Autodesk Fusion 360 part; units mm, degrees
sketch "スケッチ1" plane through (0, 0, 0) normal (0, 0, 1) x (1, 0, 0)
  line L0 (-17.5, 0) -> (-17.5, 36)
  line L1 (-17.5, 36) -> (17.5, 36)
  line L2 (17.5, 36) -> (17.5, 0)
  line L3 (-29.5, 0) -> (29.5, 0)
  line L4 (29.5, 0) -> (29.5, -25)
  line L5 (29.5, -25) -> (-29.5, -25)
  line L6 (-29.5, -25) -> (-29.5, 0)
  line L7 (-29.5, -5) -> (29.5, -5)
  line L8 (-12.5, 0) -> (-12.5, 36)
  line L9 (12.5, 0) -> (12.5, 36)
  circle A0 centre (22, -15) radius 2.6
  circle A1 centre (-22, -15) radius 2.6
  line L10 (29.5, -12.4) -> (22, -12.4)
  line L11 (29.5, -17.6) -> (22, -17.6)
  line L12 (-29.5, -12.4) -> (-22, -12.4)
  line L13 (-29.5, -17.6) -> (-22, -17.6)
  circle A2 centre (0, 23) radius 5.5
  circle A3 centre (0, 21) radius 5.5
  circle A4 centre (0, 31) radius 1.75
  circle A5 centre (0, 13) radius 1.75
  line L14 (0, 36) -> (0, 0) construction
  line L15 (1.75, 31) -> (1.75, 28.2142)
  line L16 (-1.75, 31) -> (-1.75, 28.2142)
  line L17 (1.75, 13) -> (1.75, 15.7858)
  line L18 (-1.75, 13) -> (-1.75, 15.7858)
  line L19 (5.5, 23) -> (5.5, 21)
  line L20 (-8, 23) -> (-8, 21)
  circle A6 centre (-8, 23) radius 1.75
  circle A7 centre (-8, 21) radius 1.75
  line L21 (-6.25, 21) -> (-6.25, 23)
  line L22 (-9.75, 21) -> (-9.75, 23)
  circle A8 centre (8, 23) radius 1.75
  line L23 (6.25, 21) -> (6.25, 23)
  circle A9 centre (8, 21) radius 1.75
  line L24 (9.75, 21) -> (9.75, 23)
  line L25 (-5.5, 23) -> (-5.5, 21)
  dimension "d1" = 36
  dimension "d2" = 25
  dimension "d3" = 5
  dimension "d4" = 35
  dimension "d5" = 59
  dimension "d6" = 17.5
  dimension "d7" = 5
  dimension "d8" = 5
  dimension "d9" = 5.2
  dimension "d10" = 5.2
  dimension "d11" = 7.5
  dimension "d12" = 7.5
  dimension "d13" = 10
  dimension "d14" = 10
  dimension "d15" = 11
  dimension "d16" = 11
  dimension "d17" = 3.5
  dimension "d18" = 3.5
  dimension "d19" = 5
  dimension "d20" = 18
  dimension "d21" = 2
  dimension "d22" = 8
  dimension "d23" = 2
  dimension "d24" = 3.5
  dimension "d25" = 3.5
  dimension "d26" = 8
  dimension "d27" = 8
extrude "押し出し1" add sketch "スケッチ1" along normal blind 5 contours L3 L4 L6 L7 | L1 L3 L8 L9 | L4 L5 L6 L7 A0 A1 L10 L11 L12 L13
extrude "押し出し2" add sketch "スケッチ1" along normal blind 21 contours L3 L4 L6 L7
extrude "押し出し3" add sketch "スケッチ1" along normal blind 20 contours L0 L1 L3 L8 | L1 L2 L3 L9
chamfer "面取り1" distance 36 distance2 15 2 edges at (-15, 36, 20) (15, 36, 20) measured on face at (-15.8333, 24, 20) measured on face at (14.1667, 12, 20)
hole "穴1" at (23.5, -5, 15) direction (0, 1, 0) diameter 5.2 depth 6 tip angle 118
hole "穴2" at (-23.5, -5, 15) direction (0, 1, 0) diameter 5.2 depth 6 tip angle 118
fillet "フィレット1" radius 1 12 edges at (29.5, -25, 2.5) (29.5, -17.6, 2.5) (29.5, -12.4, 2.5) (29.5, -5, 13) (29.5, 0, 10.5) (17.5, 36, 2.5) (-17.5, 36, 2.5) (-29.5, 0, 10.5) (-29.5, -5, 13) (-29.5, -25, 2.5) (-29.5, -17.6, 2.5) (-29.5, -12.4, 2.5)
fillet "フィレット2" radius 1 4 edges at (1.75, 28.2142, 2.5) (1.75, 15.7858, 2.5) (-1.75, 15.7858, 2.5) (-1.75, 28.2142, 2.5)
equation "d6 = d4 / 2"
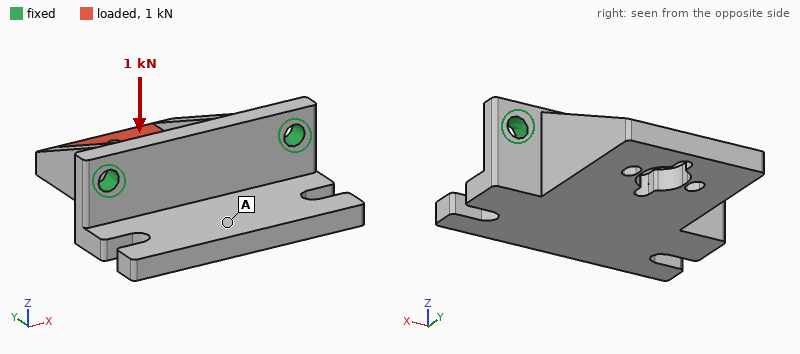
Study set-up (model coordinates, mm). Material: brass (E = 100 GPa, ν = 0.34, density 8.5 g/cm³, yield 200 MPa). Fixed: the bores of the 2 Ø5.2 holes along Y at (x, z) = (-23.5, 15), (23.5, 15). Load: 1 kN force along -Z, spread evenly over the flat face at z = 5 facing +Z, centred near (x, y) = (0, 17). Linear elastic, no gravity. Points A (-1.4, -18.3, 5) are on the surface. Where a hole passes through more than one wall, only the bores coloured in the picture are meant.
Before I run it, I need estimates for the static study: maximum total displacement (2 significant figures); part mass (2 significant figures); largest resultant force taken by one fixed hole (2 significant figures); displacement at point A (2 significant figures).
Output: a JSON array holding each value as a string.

["0.11 mm", "170 g", "580 N", "0.036 mm"]
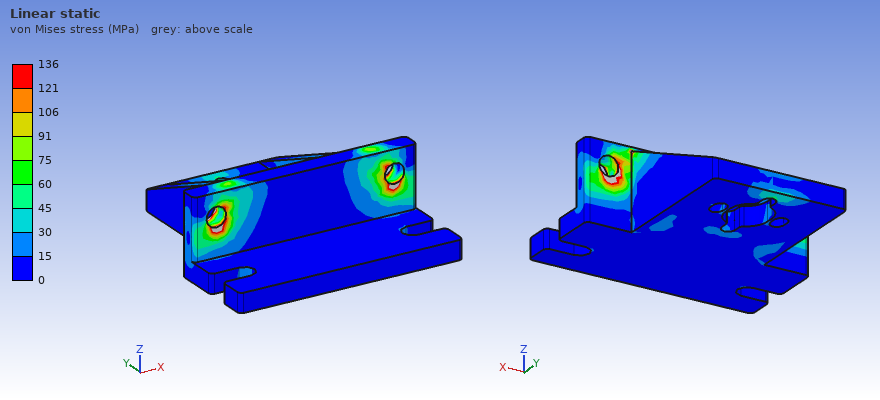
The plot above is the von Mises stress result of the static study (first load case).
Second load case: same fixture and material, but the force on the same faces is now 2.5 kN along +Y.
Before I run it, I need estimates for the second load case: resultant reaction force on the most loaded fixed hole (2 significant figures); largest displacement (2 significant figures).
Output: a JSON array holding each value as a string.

["1.3 kN", "88 µm"]
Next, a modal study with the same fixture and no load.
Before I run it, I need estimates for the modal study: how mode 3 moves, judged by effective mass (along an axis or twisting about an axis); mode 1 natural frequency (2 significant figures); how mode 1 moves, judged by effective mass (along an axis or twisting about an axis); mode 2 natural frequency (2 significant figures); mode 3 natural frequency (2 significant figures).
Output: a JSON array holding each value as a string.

["along Z", "2000 Hz", "along Y", "4000 Hz", "4800 Hz"]
